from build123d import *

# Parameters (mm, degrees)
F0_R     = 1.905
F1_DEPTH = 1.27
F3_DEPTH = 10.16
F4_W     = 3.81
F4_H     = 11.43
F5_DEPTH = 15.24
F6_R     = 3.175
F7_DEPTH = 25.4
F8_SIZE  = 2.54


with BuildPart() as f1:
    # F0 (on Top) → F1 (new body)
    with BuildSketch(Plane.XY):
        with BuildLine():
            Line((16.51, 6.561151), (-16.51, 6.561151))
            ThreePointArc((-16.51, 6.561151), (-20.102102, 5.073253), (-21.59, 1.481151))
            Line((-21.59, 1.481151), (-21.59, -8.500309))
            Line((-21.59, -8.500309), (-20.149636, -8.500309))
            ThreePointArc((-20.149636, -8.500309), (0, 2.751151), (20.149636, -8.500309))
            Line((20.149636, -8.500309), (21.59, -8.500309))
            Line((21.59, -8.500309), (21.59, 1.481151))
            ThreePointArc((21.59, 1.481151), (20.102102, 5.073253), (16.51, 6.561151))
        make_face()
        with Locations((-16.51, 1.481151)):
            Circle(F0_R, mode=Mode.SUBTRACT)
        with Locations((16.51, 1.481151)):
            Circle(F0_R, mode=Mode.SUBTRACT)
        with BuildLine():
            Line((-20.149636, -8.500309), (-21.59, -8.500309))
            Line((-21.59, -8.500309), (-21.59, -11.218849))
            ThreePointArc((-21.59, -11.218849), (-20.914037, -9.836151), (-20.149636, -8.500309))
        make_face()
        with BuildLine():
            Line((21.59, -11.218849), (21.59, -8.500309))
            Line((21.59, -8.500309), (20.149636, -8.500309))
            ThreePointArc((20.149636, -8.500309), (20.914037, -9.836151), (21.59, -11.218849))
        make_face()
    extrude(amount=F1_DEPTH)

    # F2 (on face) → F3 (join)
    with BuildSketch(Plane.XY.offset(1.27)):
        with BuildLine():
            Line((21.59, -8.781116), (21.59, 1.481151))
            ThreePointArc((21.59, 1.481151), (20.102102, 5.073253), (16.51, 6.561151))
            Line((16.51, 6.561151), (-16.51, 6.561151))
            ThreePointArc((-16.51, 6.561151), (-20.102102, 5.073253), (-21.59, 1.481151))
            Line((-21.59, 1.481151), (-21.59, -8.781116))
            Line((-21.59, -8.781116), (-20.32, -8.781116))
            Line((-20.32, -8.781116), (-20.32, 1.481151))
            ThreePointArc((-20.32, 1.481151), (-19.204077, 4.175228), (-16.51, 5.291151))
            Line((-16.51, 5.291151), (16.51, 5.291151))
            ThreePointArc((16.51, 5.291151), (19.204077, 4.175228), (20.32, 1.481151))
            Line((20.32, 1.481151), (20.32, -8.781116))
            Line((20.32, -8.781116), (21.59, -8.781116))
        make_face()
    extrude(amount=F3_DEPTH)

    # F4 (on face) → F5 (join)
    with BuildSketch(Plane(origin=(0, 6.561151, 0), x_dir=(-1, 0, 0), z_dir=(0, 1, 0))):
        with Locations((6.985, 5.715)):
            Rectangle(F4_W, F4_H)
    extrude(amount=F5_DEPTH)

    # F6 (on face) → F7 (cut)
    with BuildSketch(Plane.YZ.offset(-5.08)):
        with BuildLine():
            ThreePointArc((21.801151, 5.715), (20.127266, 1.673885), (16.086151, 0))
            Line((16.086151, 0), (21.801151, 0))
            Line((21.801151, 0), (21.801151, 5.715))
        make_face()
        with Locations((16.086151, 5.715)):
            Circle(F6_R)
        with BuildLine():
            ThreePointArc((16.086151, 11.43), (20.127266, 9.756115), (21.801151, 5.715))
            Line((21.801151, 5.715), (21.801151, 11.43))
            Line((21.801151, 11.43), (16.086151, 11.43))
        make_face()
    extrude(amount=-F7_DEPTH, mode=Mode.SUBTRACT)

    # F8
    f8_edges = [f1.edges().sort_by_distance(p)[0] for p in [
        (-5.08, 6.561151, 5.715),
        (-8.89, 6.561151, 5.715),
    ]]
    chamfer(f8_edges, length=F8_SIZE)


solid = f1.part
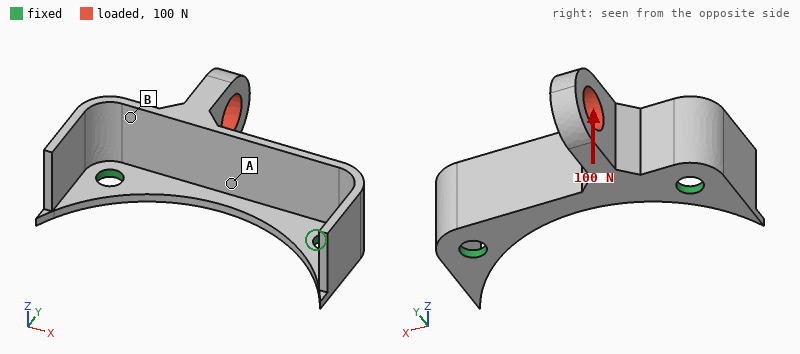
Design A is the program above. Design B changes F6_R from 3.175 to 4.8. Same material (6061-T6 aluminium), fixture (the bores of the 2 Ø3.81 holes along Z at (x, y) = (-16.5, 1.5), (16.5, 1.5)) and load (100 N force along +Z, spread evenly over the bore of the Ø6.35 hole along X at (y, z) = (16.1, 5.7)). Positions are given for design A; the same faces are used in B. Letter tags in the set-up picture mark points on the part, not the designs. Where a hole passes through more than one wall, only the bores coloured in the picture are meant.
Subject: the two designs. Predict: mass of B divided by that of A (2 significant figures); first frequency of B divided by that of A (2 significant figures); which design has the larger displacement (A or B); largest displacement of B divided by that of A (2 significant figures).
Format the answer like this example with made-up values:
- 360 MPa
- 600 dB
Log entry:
- 0.91
- 1.2
- B
- 1.1
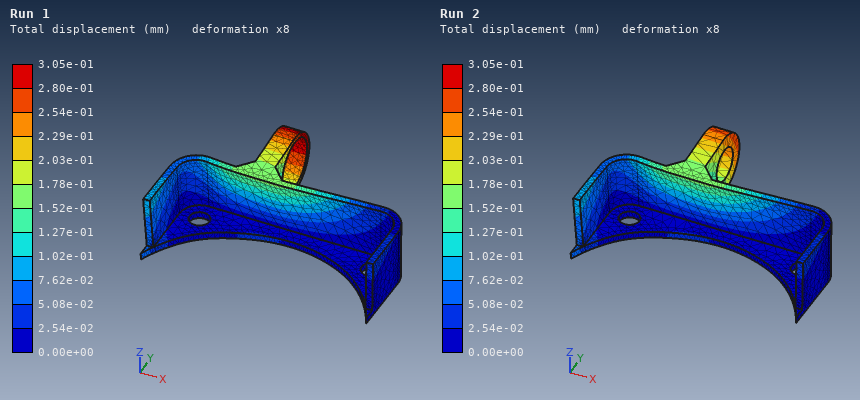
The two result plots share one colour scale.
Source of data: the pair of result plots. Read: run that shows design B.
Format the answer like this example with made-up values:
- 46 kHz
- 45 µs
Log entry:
- Run 1
